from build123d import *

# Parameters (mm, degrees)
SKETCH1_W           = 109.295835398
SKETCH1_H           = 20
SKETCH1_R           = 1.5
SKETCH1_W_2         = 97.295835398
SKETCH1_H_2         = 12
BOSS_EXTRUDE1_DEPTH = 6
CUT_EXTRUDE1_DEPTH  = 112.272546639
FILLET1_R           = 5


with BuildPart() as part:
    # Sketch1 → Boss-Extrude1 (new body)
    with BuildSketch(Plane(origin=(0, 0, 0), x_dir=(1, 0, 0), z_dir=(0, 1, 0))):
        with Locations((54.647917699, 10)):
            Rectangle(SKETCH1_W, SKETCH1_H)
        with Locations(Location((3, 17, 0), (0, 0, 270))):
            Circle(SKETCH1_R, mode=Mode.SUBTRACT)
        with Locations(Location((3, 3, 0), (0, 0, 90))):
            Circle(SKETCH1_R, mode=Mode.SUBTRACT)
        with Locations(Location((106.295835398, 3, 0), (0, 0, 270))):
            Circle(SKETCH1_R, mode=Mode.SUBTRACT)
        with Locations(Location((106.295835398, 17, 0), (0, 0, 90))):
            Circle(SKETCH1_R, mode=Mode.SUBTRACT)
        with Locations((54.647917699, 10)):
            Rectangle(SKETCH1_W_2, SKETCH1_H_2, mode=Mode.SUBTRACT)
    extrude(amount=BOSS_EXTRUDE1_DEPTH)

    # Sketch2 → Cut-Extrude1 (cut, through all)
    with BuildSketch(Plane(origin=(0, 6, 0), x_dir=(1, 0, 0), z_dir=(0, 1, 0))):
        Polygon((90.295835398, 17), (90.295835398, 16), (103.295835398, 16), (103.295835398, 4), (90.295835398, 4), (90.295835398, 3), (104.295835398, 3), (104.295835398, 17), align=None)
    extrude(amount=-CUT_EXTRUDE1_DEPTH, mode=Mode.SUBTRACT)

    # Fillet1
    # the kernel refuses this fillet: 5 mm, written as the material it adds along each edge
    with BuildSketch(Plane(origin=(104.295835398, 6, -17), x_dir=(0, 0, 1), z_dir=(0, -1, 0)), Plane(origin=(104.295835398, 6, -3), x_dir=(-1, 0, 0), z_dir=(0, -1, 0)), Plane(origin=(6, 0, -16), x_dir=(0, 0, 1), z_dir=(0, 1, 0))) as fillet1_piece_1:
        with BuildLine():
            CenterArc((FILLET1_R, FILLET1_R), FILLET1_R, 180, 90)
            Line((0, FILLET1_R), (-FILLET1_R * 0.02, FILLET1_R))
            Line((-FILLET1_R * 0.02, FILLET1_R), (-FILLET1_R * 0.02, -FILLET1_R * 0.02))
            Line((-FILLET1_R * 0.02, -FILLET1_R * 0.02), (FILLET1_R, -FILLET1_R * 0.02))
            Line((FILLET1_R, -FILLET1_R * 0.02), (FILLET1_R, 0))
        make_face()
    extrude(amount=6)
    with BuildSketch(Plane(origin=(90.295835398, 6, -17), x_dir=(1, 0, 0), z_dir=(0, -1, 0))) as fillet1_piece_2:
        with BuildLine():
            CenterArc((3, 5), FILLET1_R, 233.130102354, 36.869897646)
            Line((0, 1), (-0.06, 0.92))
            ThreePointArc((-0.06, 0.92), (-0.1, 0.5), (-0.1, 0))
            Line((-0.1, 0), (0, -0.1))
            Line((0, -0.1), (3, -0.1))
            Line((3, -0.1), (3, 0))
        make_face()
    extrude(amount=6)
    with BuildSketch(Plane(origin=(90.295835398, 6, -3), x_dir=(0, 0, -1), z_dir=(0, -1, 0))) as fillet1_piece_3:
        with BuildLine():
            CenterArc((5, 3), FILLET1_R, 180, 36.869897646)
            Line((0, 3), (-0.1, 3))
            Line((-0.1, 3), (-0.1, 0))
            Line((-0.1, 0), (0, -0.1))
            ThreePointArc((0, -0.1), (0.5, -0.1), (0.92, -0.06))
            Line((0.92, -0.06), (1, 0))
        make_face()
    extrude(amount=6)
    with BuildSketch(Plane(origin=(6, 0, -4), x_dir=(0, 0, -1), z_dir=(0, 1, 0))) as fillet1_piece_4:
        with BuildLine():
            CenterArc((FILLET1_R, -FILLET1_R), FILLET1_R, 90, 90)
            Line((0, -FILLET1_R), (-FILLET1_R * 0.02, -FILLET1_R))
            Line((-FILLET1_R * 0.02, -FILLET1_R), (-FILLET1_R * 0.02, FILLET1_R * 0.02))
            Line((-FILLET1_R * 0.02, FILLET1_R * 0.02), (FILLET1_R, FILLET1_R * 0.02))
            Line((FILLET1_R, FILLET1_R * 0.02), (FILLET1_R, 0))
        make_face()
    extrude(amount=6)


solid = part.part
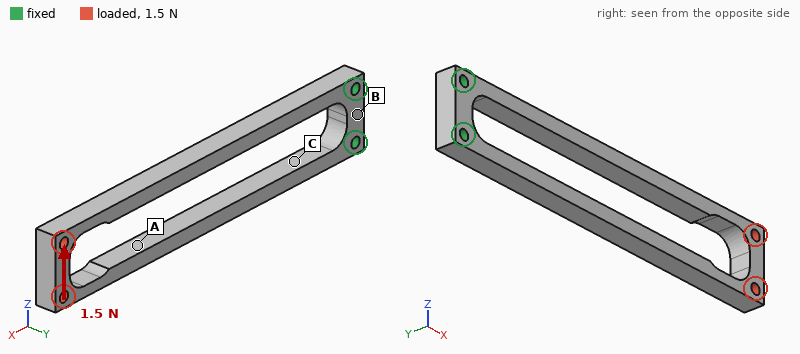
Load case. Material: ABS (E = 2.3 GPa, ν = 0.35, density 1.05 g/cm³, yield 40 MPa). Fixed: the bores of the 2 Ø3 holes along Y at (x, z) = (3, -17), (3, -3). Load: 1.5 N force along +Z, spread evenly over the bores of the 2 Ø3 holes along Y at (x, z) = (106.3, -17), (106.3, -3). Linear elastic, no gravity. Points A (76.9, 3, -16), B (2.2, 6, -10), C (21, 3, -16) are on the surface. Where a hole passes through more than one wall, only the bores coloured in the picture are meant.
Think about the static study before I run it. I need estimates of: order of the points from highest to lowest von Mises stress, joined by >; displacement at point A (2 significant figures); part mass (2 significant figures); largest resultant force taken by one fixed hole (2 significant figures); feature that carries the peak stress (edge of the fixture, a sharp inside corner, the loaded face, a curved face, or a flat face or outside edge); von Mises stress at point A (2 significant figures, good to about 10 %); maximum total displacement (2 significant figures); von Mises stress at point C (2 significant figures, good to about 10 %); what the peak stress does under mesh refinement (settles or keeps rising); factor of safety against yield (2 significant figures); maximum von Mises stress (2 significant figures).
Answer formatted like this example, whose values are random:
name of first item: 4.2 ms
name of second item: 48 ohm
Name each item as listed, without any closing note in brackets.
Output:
order of the points from highest to lowest von Mises stress, joined by >: C > A > B
displacement at point A: 0.84 mm
part mass: 6.1 g
largest resultant force taken by one fixed hole: 7.6 N
feature that carries the peak stress: a curved face
von Mises stress at point A: 0.81 MPa
maximum total displacement: 1.1 mm
von Mises stress at point C: 1.8 MPa
what the peak stress does under mesh refinement: settles
factor of safety against yield: 11
maximum von Mises stress: 3.7 MPa
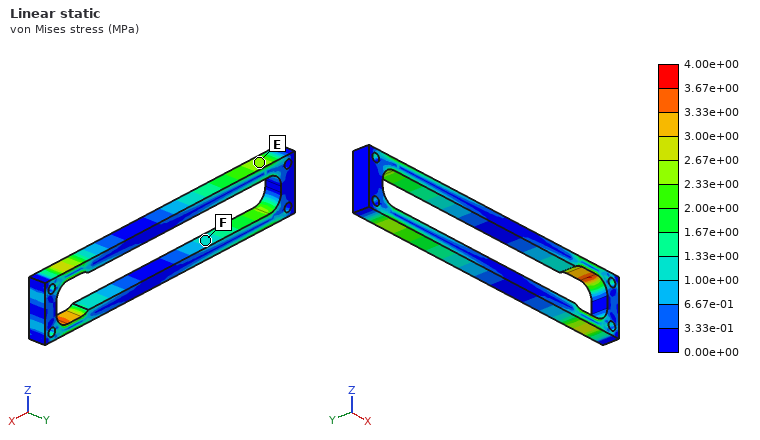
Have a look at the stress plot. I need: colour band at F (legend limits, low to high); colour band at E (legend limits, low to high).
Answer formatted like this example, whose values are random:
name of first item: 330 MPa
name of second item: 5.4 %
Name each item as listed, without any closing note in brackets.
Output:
colour band at F: 1.00e+00 to 1.33e+00 MPa
colour band at E: 2.33e+00 to 2.67e+00 MPa
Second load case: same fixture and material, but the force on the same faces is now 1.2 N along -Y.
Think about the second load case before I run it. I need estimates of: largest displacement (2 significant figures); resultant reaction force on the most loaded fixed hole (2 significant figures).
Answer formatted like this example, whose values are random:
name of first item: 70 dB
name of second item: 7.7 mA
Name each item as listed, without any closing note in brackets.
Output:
largest displacement: 1.3 mm
resultant reaction force on the most loaded fixed hole: 0.60 N
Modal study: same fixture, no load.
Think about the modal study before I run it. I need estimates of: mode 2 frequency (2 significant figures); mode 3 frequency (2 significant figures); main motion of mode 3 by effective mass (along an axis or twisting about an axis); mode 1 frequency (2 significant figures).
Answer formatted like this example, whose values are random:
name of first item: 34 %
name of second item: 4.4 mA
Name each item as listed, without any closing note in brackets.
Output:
mode 2 frequency: 130 Hz
mode 3 frequency: 480 Hz
main motion of mode 3 by effective mass: twisting about X
mode 1 frequency: 120 Hz
